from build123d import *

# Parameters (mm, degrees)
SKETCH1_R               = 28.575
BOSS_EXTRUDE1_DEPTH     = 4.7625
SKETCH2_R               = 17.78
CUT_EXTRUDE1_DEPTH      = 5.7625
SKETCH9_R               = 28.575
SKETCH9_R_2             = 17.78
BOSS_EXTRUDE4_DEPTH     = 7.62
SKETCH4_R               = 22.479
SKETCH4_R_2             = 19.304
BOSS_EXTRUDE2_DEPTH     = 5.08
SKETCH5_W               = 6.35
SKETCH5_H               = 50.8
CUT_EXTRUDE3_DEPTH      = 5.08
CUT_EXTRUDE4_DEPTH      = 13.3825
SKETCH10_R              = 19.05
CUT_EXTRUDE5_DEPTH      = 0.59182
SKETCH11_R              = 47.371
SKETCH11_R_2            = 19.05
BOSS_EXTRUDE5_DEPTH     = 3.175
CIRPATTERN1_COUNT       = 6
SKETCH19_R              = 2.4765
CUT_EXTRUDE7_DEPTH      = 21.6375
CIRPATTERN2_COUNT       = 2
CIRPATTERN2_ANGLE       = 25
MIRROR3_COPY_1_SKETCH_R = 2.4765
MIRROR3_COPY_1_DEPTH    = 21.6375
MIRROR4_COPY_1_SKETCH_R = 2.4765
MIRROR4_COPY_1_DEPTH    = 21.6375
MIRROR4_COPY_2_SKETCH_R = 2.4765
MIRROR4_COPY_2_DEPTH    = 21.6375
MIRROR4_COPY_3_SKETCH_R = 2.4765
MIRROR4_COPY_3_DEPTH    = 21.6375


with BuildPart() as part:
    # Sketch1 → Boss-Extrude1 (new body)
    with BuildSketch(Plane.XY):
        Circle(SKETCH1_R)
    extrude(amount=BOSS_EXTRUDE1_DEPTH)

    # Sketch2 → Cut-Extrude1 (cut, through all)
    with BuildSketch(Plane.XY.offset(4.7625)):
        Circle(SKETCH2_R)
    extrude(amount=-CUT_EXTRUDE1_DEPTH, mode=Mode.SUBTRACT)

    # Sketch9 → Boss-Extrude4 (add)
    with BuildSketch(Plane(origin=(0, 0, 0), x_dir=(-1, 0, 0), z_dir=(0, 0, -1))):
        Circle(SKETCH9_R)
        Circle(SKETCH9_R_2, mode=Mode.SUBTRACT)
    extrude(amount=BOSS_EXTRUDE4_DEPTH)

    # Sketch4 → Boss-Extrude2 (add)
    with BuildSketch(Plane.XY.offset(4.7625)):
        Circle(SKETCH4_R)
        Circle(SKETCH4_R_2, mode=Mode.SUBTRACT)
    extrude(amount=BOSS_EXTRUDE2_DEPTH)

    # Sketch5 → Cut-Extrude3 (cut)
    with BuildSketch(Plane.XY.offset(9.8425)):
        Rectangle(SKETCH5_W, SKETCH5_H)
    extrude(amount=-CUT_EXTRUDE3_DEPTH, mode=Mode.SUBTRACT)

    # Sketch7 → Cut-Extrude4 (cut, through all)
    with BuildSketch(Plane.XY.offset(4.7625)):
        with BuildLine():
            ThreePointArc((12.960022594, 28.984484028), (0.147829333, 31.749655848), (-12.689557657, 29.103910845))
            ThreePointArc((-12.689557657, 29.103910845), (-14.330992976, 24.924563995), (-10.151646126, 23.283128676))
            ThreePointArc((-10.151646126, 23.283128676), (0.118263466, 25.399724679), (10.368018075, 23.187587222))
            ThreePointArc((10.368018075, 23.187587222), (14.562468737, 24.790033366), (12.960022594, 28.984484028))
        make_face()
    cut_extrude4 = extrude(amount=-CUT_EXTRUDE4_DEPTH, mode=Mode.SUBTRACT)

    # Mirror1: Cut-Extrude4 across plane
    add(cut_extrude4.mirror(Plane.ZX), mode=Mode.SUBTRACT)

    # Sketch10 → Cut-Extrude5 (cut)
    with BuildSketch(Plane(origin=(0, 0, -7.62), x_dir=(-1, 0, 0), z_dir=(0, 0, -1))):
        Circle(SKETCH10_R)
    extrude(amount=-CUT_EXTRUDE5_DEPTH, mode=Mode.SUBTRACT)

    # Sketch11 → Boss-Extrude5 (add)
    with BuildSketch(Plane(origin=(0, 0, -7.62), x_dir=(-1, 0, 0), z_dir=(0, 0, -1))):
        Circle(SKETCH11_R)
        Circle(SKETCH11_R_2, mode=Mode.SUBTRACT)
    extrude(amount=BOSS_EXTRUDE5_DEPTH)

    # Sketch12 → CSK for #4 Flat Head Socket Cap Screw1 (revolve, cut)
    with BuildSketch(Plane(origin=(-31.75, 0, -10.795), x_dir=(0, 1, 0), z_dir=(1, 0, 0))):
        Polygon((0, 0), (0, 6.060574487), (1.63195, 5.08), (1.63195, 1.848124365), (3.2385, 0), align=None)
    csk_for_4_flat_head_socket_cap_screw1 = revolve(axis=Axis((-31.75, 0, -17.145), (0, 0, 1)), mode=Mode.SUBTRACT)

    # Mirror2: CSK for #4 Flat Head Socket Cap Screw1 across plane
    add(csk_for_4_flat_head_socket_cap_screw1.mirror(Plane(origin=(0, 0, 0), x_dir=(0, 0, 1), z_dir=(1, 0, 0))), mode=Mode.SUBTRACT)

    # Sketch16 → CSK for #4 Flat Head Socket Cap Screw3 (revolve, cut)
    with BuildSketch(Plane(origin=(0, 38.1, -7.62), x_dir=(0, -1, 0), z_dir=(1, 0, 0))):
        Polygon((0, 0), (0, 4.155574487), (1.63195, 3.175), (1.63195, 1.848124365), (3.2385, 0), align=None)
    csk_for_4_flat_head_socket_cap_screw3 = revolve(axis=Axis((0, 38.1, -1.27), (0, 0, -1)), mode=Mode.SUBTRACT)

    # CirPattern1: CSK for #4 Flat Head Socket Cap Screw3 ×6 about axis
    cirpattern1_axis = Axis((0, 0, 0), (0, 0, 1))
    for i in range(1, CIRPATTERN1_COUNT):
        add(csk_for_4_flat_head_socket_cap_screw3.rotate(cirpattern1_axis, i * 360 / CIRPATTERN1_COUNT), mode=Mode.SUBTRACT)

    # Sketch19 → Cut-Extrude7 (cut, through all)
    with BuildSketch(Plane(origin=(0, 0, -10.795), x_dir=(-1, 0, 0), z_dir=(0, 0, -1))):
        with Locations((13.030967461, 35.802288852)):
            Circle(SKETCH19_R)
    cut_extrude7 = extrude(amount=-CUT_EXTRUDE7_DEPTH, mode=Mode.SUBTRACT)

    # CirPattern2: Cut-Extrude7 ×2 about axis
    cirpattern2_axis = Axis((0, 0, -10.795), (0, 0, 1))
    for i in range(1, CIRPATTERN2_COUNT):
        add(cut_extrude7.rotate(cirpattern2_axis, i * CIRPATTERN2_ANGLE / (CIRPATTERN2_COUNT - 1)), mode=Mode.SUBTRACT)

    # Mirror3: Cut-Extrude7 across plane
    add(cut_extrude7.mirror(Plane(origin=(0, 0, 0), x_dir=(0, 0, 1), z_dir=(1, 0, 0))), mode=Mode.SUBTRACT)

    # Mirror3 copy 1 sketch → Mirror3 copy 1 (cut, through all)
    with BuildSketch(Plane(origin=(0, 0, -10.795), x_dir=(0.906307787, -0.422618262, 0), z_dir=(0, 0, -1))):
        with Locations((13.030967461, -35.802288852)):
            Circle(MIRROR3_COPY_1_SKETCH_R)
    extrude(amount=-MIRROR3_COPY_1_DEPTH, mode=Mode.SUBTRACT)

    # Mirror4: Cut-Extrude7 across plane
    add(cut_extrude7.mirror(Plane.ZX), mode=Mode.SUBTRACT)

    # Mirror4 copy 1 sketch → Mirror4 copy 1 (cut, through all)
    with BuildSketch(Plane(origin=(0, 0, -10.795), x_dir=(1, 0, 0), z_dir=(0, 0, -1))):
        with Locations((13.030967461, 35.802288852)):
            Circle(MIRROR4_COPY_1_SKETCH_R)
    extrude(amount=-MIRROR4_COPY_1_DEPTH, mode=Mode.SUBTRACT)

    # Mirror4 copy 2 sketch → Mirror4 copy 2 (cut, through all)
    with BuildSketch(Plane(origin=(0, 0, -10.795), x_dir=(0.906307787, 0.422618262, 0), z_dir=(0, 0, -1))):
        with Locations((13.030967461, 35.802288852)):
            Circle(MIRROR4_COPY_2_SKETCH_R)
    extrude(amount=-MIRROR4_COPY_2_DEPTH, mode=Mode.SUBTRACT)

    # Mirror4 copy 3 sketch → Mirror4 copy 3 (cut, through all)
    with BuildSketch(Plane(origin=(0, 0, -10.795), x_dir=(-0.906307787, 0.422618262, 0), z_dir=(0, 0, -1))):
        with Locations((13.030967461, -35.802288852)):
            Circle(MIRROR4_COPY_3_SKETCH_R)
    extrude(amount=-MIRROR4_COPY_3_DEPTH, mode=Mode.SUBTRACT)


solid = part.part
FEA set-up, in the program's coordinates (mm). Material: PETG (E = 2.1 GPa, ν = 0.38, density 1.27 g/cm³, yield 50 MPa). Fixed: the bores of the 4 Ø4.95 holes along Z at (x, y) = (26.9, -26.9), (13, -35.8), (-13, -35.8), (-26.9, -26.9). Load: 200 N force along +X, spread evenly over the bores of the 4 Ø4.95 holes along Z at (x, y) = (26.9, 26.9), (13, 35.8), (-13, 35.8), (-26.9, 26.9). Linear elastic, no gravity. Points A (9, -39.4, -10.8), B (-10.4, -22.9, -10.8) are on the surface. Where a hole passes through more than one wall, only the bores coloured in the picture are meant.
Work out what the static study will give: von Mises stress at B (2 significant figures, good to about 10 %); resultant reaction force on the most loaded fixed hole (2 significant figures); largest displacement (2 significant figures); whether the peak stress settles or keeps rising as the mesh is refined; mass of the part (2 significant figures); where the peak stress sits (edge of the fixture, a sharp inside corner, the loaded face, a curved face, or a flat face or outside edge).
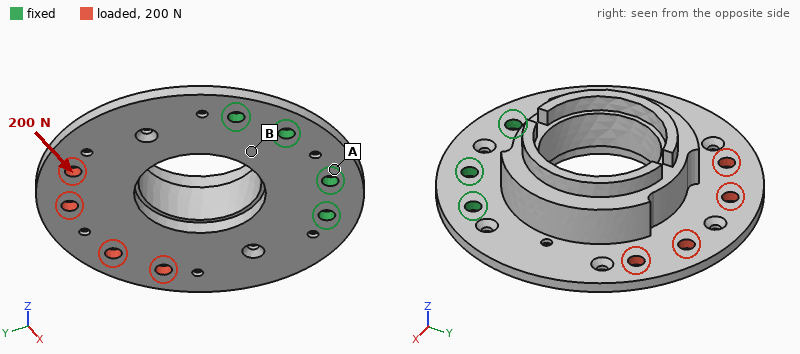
3.1 MPa
220 N
0.32 mm
keeps rising
47 g
edge of the fixture
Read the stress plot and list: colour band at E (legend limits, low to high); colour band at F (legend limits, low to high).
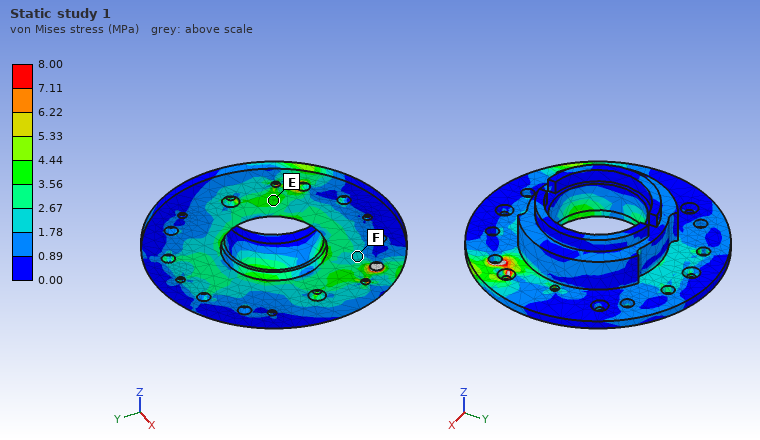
3.56 to 4.44 MPa
1.78 to 2.67 MPa
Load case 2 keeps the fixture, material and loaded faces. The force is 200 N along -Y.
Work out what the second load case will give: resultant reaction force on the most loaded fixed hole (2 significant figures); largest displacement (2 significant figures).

82 N
0.14 mm
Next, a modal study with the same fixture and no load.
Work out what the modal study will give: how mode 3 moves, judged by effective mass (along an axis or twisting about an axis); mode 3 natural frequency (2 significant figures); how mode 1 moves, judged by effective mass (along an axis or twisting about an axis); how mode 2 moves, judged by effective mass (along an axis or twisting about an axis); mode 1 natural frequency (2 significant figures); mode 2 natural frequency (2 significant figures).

along X
1200 Hz
along Z
twisting about Y
190 Hz
730 Hz
